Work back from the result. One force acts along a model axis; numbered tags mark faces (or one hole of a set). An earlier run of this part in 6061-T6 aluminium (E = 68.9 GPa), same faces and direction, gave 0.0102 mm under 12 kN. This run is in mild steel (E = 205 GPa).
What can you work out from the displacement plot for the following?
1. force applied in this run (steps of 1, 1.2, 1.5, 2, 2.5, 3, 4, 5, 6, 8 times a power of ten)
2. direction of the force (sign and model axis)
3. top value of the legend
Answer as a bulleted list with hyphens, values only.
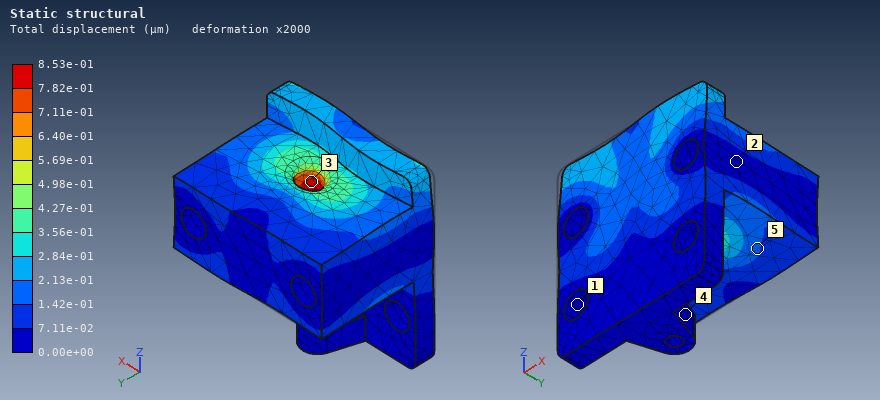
- 3 kN
- +X
- 8.53e-01 µm
